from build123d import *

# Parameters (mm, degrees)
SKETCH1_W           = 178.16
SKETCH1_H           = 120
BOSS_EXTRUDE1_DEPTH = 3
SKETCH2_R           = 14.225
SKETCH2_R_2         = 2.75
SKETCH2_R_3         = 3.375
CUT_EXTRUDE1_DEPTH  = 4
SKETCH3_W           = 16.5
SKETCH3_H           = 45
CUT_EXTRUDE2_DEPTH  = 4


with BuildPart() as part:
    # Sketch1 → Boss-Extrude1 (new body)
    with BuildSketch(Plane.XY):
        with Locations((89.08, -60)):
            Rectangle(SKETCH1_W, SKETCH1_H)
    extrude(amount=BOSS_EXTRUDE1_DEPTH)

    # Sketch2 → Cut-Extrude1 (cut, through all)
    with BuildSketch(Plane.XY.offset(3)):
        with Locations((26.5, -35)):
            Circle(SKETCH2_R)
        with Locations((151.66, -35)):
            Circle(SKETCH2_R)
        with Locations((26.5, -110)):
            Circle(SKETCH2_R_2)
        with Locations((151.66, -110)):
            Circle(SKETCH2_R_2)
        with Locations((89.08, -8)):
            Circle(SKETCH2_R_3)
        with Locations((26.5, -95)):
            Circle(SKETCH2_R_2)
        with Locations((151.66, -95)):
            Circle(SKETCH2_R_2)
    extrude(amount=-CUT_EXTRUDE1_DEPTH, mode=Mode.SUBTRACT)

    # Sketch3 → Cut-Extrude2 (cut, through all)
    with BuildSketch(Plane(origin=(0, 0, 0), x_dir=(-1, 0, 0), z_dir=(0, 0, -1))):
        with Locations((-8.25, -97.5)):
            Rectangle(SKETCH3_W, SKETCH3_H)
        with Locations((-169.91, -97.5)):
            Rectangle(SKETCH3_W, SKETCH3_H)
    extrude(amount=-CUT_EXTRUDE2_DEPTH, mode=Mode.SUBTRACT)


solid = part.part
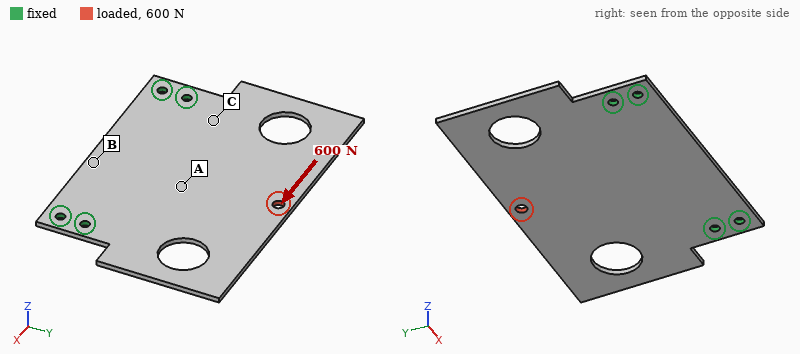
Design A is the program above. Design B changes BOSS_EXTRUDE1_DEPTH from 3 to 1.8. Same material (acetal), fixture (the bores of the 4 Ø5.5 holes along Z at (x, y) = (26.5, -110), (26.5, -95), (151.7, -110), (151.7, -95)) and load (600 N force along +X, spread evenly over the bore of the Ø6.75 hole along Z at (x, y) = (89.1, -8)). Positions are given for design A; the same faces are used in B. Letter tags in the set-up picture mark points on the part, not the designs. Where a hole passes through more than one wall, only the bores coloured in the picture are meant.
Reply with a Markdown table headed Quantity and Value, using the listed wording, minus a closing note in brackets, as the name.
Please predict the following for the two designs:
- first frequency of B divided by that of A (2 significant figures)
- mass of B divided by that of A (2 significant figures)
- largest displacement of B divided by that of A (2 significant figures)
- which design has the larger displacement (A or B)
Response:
| Quantity | Value |
|---|---|
| first frequency of B divided by that of A | 0.61 |
| mass of B divided by that of A | 0.60 |
| largest displacement of B divided by that of A | 1.7 |
| which design has the larger displacement | B |
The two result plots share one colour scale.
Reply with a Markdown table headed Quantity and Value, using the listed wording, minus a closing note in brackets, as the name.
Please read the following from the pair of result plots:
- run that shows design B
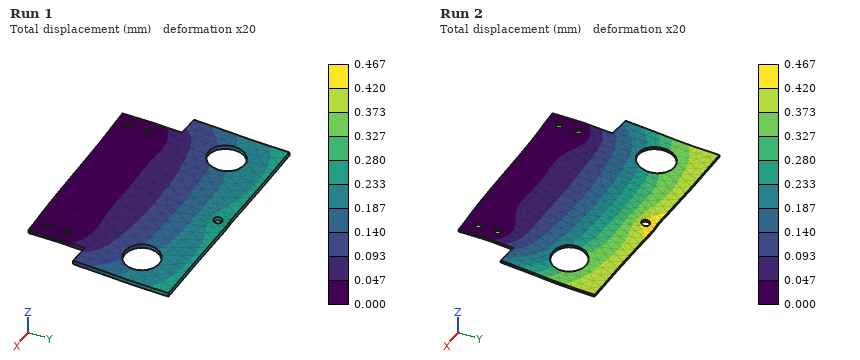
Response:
| Quantity | Value |
|---|---|
| run that shows design B | Run 2 |
